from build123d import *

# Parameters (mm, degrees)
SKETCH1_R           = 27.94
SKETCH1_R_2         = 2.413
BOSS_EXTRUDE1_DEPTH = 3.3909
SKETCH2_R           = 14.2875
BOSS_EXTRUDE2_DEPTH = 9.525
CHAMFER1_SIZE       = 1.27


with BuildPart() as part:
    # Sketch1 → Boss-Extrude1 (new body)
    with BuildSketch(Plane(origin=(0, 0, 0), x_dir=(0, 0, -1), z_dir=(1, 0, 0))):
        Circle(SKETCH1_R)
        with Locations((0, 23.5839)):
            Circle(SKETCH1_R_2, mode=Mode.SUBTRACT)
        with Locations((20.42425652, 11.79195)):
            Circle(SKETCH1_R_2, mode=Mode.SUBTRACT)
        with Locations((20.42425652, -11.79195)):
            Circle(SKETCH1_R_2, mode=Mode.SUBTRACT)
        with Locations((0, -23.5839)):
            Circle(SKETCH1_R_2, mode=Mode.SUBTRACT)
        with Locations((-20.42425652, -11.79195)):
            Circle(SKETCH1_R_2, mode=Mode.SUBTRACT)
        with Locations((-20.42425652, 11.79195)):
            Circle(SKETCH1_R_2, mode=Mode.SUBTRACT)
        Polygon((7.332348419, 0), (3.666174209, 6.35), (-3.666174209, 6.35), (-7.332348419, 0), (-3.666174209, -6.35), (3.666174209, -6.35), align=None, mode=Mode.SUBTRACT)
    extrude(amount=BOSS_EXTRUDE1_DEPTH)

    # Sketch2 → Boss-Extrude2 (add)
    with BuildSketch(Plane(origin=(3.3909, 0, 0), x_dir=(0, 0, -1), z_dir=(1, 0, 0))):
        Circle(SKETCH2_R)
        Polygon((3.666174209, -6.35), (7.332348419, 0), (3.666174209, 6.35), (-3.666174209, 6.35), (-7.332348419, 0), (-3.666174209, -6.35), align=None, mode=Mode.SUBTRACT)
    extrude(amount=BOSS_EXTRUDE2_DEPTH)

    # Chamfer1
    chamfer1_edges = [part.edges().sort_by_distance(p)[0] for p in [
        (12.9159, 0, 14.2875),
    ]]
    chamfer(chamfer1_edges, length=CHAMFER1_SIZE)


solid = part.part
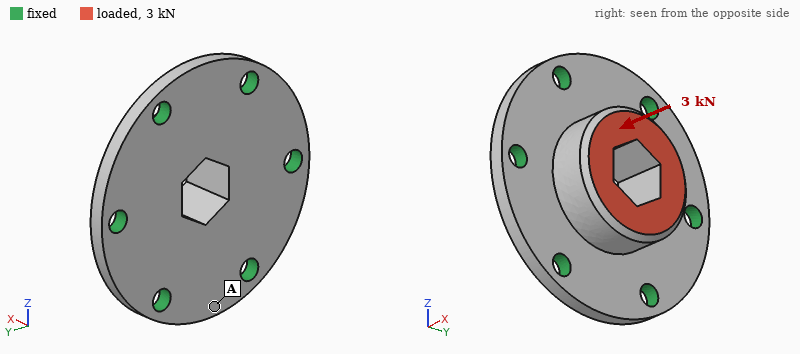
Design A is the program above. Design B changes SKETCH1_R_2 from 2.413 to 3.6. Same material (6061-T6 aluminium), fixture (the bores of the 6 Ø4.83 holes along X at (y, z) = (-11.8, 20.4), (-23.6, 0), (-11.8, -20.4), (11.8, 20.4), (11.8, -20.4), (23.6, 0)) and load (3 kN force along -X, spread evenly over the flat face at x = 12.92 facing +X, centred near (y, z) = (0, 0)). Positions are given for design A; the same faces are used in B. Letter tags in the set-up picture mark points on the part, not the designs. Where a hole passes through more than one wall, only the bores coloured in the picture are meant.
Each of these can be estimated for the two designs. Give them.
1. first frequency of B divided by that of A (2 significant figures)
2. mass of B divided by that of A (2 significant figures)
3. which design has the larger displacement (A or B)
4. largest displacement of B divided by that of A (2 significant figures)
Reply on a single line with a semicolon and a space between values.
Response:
1.2; 0.96; A; 0.72
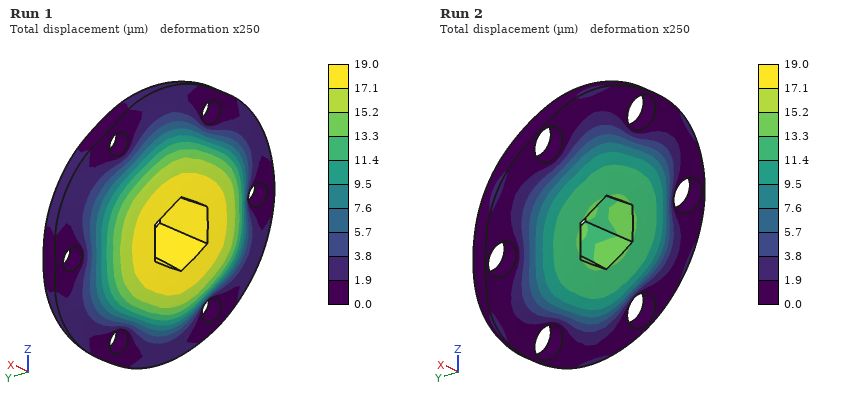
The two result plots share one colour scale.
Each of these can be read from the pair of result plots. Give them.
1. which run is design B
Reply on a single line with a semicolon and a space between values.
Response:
Run 2
